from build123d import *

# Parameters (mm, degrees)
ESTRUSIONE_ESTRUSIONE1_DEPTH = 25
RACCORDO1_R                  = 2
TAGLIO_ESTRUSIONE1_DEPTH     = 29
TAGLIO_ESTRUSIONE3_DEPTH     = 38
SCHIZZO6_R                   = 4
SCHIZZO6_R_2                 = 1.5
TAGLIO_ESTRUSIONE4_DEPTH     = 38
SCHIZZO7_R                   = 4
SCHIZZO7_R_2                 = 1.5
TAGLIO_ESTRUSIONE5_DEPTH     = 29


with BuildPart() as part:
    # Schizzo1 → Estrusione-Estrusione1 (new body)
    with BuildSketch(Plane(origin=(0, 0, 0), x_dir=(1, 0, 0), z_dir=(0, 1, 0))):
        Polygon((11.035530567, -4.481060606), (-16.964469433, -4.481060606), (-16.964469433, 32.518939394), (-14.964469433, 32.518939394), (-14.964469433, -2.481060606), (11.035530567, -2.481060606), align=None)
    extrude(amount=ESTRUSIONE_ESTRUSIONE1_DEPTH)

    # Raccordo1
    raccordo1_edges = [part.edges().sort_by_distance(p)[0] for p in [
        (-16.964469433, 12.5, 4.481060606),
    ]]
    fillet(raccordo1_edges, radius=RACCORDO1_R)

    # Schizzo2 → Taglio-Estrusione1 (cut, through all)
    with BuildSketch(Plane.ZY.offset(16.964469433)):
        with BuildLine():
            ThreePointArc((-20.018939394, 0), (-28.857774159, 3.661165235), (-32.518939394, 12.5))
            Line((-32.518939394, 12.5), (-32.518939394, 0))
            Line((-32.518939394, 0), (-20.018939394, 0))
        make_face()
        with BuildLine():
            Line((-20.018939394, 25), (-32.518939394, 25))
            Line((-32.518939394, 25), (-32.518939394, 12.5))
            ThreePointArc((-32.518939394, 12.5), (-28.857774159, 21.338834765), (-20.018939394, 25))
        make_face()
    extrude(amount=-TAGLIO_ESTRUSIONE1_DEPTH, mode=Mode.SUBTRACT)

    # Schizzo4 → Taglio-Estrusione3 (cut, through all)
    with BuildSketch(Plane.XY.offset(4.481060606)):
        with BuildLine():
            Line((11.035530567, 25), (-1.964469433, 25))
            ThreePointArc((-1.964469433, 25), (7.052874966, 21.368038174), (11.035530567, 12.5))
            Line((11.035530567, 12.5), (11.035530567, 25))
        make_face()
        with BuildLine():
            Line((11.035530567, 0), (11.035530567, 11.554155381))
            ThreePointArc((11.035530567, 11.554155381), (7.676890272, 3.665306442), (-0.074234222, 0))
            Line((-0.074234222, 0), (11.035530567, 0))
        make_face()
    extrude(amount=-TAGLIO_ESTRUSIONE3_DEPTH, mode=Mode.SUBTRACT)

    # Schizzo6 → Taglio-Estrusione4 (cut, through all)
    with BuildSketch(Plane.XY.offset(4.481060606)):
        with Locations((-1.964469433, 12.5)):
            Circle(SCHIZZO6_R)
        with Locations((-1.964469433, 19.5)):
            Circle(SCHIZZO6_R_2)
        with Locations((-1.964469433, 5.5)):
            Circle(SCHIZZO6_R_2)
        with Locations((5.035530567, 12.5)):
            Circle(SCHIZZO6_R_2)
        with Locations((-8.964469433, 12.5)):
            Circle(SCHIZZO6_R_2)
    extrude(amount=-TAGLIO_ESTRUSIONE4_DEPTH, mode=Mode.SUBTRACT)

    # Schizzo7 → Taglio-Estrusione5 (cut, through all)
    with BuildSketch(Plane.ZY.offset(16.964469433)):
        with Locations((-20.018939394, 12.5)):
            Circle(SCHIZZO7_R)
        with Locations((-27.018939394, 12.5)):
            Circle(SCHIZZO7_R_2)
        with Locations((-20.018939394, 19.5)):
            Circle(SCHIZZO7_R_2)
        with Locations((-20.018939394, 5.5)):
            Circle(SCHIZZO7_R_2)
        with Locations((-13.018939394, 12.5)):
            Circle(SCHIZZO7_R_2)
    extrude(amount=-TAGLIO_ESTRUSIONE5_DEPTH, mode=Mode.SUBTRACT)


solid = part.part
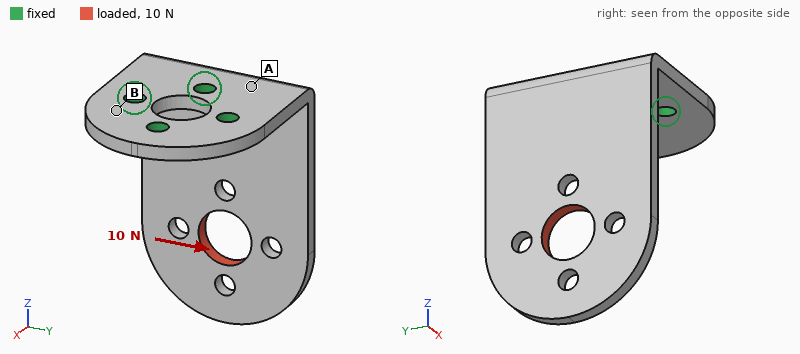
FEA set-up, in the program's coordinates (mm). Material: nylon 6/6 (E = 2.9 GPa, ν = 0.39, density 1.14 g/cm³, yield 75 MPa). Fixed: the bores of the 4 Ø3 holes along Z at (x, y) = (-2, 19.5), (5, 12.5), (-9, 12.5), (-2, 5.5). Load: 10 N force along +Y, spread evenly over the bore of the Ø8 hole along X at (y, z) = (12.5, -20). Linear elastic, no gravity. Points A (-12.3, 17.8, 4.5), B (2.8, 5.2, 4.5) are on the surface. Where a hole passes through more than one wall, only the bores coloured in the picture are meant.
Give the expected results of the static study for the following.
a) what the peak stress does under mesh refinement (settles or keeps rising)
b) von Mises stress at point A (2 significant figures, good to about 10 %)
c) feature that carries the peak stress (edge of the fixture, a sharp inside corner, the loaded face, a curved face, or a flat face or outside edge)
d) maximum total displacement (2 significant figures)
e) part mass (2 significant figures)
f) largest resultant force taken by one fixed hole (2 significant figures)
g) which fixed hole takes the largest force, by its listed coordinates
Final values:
keeps rising
4.2 MPa
edge of the fixture
0.59 mm
2.9 g
9.3 N
(-9, 12.5)
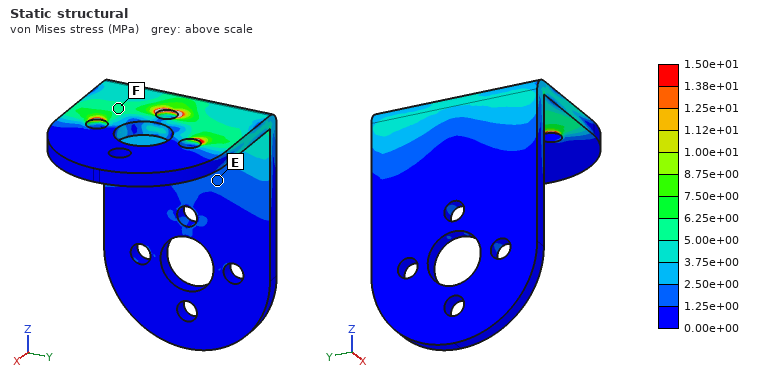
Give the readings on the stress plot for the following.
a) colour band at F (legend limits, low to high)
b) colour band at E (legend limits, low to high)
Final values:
5.00e+00 to 6.25e+00 MPa
1.25e+00 to 2.50e+00 MPa
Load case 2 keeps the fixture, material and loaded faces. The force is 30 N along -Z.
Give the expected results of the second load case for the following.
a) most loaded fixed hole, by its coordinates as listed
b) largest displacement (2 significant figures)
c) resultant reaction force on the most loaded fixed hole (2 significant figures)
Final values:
(-9, 12.5)
0.58 mm
36 N
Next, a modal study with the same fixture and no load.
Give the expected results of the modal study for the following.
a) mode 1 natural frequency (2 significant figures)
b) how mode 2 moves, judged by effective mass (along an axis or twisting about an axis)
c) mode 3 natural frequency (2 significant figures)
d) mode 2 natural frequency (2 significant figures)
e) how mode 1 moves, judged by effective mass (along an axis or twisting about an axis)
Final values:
380 Hz
along Y
1400 Hz
710 Hz
along X
